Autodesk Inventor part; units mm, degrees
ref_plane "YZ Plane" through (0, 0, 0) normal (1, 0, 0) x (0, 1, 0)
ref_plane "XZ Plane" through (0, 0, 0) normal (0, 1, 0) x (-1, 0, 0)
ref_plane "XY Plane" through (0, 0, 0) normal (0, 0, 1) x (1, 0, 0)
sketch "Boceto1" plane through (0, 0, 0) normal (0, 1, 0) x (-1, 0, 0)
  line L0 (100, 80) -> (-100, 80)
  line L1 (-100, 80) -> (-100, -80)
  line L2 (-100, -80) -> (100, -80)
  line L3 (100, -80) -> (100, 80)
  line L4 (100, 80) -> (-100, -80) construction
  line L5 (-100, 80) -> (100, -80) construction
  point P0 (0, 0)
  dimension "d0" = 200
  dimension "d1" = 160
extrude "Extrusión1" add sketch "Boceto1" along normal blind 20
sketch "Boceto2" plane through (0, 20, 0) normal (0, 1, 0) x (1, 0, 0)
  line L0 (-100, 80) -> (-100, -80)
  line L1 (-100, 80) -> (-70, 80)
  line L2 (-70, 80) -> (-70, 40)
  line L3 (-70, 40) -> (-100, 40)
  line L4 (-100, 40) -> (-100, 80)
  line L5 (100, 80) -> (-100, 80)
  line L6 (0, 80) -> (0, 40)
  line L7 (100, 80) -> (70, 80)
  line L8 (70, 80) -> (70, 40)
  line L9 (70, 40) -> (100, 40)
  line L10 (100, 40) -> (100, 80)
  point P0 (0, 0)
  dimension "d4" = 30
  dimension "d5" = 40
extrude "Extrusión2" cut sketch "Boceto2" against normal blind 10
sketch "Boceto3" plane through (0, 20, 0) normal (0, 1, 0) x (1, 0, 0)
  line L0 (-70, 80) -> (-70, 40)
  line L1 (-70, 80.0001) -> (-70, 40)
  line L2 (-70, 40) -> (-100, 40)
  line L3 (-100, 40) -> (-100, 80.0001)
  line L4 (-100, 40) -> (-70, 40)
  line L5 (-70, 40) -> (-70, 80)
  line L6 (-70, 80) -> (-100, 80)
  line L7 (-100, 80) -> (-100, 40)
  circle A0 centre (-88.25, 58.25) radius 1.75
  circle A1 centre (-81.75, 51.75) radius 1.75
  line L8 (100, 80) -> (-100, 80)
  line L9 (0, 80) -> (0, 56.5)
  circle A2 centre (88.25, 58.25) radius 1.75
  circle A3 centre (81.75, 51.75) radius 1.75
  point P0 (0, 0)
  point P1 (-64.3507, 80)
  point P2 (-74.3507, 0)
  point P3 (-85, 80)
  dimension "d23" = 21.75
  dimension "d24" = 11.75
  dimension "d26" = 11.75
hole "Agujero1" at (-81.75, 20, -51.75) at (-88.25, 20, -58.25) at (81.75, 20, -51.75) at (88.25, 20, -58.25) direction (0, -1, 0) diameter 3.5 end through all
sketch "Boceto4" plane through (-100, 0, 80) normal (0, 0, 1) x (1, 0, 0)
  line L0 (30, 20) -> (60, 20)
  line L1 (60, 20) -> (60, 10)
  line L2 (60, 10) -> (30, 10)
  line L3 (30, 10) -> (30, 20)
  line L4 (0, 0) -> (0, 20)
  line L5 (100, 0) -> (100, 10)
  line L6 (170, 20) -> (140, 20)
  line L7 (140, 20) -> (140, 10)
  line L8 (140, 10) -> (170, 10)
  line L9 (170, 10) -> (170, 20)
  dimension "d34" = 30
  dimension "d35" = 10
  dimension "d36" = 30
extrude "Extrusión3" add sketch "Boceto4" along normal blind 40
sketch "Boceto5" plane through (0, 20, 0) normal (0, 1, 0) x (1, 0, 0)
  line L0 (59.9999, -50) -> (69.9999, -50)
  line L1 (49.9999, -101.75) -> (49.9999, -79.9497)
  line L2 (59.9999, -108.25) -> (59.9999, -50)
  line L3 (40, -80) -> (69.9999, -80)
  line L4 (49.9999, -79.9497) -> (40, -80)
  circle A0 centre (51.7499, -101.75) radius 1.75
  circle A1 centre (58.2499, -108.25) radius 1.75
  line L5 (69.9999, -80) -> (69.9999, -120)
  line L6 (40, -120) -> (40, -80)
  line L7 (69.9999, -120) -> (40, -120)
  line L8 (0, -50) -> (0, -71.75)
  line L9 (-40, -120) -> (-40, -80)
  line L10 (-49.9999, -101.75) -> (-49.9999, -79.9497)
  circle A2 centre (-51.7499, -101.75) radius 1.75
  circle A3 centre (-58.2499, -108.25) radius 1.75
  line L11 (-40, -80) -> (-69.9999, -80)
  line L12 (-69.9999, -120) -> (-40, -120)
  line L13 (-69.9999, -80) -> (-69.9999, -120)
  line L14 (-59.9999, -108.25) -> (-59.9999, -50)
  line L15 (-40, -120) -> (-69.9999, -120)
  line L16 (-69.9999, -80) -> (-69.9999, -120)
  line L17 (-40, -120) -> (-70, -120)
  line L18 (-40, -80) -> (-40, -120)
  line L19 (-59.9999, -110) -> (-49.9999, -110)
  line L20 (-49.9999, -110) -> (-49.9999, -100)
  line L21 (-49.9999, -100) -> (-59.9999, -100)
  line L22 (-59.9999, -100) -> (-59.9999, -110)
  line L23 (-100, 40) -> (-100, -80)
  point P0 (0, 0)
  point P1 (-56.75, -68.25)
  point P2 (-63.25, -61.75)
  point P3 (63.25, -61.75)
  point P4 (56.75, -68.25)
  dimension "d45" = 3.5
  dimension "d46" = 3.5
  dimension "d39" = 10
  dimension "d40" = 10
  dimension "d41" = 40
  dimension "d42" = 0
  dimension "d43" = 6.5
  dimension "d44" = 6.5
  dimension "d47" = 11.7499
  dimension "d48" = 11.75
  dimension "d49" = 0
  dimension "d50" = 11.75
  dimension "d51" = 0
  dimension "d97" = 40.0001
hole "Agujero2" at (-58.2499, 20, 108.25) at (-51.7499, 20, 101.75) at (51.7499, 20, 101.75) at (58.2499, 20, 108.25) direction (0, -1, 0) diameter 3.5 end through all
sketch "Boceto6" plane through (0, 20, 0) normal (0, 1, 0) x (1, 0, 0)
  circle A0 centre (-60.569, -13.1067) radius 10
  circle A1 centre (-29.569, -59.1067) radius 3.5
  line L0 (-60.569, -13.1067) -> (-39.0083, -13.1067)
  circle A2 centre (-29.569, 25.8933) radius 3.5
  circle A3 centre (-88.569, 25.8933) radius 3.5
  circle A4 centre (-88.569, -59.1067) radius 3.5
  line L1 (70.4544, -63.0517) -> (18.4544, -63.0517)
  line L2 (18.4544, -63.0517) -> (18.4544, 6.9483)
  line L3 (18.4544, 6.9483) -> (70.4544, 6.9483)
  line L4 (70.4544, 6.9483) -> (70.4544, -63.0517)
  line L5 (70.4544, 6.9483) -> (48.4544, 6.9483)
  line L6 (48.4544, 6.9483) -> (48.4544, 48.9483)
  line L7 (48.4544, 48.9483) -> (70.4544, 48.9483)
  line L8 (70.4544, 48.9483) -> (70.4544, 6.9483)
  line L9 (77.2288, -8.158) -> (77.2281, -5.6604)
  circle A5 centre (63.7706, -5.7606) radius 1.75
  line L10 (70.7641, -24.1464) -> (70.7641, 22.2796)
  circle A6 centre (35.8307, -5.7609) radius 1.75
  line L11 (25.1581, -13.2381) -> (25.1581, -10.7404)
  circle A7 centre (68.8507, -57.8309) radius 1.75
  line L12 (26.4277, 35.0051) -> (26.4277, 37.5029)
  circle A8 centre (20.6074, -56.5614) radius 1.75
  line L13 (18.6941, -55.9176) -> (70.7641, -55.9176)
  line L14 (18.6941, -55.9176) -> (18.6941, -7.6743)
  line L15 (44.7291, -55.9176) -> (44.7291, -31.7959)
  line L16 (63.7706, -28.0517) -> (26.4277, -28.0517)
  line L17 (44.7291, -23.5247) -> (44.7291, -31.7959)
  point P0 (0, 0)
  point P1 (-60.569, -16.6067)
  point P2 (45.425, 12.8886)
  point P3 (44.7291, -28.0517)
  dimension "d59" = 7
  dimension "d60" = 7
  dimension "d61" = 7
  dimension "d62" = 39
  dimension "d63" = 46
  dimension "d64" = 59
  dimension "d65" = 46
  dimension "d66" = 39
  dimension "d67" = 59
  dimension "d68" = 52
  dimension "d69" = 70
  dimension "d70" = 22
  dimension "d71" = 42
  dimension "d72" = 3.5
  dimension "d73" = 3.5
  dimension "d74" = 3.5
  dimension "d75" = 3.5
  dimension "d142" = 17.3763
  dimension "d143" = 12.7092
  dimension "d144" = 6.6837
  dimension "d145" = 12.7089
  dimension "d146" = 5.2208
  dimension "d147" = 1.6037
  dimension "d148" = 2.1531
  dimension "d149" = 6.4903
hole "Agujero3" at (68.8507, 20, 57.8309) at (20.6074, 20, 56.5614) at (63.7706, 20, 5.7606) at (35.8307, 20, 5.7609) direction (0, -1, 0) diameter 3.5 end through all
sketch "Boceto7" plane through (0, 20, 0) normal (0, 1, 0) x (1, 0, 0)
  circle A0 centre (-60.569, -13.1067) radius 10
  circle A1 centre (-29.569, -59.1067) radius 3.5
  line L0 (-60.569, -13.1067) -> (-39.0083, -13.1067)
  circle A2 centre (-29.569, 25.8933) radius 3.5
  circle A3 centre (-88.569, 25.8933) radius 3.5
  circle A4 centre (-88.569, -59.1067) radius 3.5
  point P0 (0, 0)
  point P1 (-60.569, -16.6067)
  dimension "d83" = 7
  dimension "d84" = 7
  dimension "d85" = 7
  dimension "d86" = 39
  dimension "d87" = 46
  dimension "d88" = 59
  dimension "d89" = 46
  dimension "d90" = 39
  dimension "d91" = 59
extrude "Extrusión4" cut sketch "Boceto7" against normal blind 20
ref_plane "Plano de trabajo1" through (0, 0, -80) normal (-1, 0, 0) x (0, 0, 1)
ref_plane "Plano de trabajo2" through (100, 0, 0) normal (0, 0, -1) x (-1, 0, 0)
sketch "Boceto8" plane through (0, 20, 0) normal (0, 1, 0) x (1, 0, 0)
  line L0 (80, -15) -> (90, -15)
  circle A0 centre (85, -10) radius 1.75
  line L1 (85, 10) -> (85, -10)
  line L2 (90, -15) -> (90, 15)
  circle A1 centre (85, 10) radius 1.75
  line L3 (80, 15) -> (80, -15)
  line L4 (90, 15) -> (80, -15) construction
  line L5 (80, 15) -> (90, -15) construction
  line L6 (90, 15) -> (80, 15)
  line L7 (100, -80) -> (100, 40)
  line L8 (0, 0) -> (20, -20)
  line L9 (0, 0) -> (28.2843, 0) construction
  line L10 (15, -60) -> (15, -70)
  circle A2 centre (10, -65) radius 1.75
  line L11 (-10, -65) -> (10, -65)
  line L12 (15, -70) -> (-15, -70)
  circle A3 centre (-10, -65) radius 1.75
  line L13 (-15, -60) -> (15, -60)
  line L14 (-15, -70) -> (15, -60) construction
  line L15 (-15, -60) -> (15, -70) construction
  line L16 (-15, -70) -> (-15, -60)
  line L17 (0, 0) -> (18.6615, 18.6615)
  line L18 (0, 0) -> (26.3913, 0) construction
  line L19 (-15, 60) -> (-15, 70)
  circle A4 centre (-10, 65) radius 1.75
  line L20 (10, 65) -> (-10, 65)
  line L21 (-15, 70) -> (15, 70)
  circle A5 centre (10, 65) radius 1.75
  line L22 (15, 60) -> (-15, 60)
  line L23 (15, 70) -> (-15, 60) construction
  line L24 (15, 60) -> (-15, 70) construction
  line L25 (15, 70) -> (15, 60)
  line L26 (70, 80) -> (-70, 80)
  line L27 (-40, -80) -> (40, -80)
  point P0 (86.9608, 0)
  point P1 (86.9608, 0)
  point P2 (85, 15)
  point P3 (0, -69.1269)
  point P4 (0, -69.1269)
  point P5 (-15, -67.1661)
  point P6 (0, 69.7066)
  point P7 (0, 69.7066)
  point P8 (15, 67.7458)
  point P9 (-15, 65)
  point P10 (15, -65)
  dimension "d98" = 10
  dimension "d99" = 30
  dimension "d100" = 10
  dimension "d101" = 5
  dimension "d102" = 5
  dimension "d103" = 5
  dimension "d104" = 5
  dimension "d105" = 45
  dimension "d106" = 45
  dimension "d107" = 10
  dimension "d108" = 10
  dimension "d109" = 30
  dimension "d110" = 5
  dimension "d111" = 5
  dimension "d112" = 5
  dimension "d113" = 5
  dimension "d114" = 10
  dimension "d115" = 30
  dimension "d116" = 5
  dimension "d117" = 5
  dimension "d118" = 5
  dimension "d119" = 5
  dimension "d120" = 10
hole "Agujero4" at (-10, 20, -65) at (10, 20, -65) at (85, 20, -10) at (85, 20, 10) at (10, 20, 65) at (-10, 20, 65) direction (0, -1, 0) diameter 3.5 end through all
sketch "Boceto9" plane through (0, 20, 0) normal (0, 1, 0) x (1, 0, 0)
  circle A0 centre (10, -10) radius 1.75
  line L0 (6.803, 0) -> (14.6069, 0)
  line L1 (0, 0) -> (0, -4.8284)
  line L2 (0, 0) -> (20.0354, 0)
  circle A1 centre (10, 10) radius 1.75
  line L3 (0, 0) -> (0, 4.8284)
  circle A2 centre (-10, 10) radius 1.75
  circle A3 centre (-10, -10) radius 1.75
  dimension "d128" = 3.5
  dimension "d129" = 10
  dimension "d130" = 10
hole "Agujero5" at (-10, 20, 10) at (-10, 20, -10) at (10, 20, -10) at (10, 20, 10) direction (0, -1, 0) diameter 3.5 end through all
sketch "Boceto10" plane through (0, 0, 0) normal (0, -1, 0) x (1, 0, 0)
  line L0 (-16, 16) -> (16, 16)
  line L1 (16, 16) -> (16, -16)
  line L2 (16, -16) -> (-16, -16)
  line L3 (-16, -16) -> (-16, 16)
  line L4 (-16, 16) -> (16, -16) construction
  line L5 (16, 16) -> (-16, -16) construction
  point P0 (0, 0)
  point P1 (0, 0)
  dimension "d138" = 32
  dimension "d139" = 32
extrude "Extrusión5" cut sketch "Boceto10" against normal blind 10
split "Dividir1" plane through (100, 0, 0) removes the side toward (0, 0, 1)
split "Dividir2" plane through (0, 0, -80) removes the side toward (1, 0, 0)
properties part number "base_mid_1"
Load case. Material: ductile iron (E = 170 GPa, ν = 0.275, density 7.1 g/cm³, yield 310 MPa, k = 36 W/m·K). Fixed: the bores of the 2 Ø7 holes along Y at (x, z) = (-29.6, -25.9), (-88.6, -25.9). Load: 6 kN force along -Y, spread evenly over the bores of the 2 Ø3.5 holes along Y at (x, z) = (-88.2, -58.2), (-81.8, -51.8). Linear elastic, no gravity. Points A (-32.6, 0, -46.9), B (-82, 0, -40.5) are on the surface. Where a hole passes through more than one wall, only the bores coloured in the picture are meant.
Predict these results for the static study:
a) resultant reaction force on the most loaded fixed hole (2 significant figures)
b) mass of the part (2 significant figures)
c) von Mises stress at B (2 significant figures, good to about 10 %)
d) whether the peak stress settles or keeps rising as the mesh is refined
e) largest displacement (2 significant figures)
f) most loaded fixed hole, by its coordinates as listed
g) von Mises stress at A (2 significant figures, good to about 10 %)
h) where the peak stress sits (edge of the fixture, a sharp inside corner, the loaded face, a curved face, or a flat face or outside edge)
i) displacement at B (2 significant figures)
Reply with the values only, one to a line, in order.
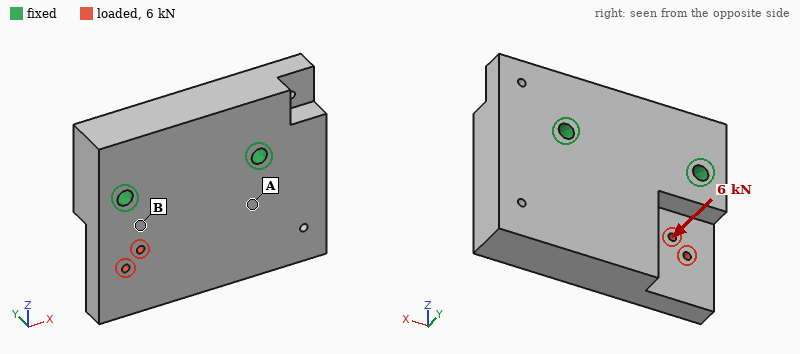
5.4 kN
1.0 kg
56 MPa
keeps rising
54 µm
(-88.6, -25.9)
14 MPa
a sharp inside corner
9.5 µm
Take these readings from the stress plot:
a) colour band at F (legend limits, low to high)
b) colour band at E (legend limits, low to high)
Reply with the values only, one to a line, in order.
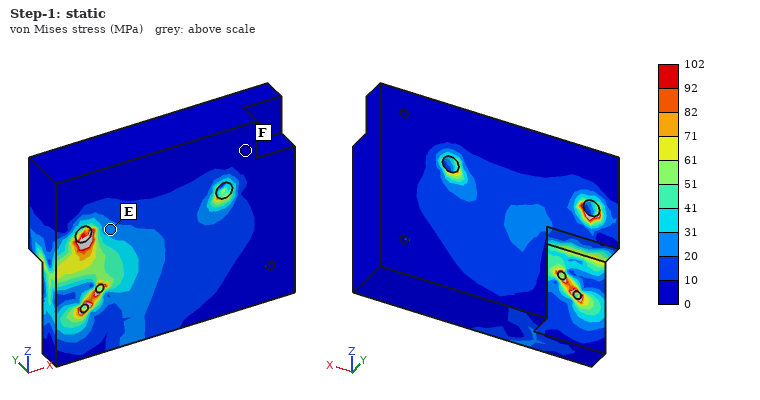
0 to 10 MPa
20 to 31 MPa
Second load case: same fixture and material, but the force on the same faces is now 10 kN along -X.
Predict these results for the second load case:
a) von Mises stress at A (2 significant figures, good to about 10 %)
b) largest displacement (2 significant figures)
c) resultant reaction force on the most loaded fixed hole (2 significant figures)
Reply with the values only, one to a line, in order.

8.7 MPa
9.5 µm
6.8 kN
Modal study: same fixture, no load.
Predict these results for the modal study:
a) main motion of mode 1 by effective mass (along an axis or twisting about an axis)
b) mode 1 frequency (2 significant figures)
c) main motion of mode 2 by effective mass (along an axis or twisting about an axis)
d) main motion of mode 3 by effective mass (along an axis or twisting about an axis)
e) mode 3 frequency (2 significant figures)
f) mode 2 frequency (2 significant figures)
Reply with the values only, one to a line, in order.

along Y
3800 Hz
twisting about Z
along X
8700 Hz
6200 Hz
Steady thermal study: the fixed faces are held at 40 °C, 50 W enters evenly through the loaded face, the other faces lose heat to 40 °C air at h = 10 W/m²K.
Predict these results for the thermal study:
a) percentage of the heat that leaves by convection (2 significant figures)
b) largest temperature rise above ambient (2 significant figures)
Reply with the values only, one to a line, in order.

7.3 %
80 K
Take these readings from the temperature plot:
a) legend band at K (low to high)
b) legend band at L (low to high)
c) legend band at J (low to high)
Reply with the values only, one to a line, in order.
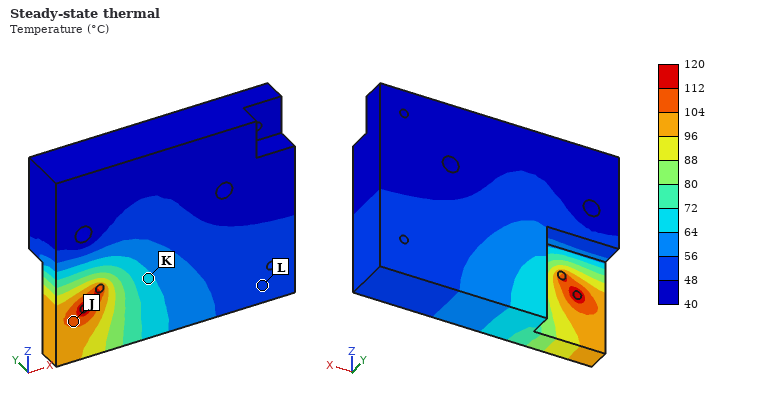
64 to 72 °C
48 to 56 °C
104 to 112 °C
